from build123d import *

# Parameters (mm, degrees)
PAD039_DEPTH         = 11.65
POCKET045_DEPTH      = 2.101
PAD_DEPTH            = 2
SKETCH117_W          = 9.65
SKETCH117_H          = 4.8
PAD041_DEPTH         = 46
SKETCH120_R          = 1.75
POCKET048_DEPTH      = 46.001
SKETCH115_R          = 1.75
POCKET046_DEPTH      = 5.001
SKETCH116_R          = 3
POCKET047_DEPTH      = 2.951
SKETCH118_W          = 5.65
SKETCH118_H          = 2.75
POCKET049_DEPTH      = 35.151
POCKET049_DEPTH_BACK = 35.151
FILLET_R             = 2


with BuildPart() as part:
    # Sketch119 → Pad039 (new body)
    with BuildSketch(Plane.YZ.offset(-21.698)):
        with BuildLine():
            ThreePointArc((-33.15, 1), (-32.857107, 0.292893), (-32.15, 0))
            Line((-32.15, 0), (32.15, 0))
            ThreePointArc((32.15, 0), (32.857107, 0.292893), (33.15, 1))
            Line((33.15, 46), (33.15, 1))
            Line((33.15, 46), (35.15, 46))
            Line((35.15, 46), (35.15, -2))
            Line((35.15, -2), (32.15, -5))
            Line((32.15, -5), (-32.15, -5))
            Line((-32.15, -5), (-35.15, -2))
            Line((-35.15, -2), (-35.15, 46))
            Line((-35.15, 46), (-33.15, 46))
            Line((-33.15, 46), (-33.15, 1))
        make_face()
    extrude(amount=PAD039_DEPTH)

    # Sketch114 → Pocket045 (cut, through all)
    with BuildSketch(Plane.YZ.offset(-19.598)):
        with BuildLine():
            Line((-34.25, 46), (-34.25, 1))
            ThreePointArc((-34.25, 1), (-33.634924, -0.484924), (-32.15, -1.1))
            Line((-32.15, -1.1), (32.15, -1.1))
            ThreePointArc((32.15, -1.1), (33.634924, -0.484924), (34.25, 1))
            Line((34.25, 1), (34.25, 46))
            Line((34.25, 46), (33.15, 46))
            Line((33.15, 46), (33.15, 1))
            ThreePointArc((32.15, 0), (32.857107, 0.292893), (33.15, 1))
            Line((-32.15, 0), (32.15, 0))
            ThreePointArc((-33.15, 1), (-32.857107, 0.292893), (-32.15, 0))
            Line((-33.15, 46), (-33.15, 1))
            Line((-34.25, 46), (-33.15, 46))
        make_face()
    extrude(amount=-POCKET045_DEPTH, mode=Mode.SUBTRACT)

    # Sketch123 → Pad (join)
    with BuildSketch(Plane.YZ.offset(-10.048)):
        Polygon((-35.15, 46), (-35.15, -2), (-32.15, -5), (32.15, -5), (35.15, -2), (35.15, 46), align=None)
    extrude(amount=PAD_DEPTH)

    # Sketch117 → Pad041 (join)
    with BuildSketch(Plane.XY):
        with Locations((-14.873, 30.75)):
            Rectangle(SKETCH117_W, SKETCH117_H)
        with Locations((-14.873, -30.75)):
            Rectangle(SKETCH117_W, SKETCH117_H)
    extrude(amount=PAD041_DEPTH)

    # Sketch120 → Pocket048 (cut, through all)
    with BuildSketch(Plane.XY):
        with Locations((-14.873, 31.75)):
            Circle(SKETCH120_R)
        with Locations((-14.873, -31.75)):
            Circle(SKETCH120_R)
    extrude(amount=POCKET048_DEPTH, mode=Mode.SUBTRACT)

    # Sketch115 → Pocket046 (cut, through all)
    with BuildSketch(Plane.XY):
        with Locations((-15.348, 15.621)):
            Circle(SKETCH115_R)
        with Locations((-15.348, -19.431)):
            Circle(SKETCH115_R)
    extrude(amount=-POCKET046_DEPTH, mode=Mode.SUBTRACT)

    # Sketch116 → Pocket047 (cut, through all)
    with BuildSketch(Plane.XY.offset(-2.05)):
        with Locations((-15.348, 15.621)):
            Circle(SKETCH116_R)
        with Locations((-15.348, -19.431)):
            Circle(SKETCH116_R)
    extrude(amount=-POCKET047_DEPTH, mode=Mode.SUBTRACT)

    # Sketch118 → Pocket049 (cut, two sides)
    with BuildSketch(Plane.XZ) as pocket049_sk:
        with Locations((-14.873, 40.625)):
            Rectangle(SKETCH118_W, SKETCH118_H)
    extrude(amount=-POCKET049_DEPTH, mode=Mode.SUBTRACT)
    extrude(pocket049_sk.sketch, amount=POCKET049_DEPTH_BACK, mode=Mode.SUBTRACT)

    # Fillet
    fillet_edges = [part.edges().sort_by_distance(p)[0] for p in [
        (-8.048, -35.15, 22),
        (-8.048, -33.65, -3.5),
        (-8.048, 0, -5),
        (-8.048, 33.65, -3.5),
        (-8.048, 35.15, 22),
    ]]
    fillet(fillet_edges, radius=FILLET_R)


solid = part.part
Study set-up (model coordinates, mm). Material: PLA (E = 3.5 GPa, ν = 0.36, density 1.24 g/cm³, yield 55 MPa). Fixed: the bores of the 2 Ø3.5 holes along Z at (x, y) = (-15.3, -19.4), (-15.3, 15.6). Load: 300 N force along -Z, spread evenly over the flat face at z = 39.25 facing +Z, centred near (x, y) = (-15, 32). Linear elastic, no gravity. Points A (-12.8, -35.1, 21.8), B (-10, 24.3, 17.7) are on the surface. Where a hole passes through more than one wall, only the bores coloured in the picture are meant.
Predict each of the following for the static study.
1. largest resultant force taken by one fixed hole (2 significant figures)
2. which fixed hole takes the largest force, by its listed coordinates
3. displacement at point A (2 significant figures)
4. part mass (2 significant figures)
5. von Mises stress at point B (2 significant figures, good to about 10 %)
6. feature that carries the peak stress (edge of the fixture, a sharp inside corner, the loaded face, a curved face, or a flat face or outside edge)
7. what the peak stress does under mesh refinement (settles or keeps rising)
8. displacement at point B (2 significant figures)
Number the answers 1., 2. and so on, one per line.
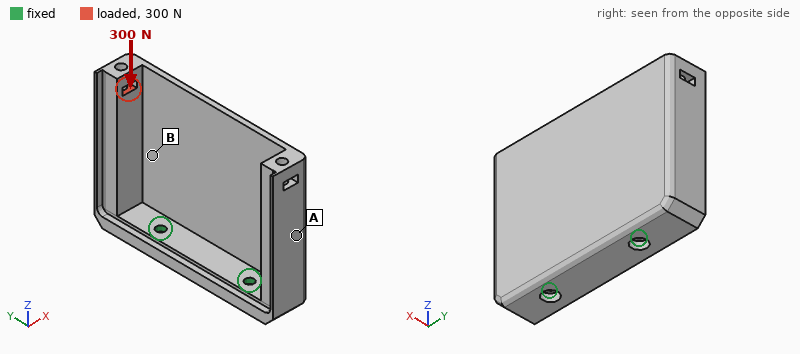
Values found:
1. 420 N
2. (-15.3, 15.6)
3. 0.28 mm
4. 20 g
5. 6.0 MPa
6. edge of the fixture
7. keeps rising
8. 0.32 mm
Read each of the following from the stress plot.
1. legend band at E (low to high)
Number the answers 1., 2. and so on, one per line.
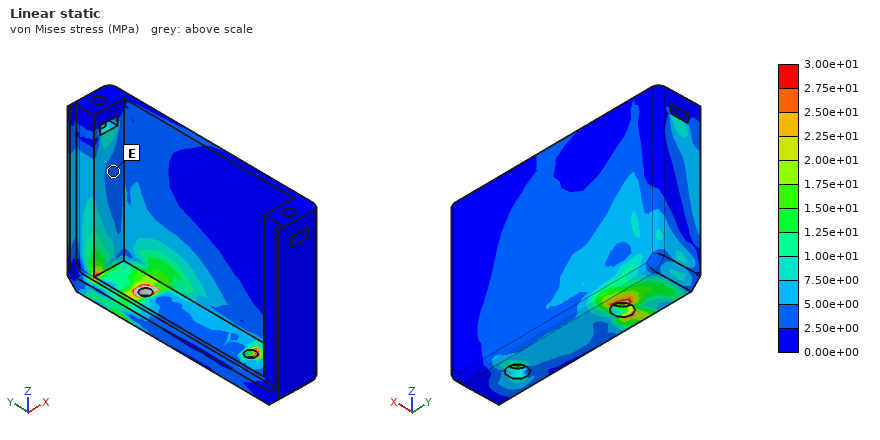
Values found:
1. 2.50e+00 to 5.00e+00 MPa
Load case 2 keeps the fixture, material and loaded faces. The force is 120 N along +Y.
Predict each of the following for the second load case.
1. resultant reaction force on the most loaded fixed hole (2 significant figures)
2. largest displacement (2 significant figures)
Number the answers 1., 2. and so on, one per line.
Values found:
1. 150 N
2. 0.96 mm
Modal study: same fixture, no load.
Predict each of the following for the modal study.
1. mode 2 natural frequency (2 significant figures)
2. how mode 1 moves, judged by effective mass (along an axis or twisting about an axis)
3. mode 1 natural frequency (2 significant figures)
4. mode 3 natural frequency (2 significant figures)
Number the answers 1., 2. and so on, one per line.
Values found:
1. 530 Hz
2. along X
3. 370 Hz
4. 1200 Hz
